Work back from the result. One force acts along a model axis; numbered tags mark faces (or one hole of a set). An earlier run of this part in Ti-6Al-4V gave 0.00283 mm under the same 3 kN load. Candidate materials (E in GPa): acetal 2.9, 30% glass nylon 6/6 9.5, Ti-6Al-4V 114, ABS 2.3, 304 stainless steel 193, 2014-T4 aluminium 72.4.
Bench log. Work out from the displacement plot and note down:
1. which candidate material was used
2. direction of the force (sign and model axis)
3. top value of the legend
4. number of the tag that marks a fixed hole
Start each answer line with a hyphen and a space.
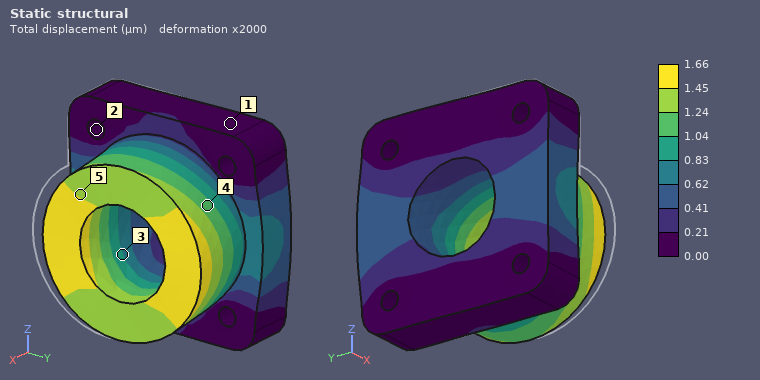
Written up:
- 304 stainless steel
- +Y
- 1.66 µm
- 2
